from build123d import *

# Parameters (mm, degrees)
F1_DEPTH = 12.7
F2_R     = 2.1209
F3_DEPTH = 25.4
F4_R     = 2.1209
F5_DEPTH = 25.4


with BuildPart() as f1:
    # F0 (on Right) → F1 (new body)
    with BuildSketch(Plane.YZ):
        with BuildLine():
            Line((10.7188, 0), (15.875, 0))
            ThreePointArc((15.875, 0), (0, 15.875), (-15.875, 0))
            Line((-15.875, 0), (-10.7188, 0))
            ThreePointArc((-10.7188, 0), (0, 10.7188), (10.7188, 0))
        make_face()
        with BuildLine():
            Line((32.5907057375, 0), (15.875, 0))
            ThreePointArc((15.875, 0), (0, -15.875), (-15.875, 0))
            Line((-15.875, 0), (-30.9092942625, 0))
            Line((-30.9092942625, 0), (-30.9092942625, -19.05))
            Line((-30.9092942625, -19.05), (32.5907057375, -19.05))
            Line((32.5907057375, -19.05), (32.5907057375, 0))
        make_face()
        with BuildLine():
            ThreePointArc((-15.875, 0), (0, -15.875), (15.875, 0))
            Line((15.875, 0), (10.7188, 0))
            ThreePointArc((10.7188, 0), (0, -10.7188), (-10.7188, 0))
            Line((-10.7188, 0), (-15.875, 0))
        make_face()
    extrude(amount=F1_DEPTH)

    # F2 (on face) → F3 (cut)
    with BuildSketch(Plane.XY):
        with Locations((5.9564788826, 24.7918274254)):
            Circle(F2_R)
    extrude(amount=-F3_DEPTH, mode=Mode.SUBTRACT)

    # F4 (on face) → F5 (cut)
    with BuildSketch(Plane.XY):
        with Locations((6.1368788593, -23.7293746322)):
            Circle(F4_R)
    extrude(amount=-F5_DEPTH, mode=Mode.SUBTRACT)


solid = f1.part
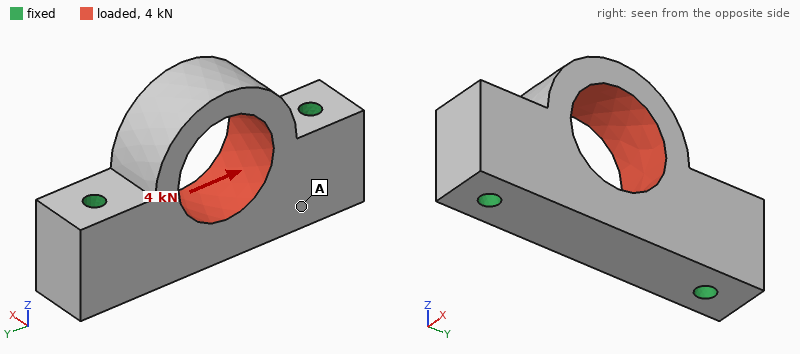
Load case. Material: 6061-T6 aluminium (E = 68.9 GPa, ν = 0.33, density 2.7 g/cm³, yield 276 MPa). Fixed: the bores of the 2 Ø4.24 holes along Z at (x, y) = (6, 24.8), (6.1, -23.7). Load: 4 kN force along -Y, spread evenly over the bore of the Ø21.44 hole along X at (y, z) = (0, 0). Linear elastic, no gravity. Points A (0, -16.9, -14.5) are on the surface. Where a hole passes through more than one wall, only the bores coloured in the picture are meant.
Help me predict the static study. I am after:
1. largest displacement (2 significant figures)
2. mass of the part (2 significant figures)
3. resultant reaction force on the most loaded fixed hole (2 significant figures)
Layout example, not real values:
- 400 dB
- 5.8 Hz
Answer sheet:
- 23 µm
- 41 g
- 2.1 kN
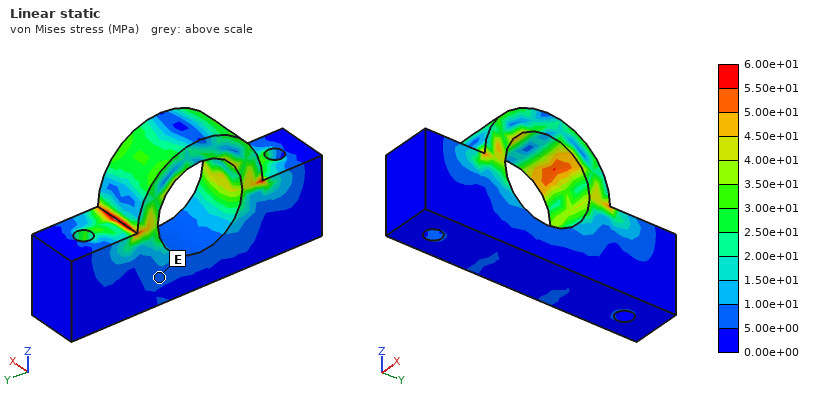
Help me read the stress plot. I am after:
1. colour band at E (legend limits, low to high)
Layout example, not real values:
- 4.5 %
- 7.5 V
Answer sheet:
- 5.00e+00 to 1.00e+01 MPa
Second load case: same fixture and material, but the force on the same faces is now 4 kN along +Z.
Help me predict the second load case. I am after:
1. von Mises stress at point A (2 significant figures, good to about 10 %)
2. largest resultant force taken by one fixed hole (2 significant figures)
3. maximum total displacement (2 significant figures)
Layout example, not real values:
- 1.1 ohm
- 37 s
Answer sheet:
- 11 MPa
- 2.0 kN
- 10 µm
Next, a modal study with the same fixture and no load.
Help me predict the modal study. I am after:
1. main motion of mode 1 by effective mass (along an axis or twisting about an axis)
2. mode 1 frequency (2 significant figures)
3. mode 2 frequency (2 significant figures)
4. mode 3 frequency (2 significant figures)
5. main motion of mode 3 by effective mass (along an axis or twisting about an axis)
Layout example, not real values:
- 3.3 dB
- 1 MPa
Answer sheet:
- along X
- 11 kHz
- 19 kHz
- 19 kHz
- along X
